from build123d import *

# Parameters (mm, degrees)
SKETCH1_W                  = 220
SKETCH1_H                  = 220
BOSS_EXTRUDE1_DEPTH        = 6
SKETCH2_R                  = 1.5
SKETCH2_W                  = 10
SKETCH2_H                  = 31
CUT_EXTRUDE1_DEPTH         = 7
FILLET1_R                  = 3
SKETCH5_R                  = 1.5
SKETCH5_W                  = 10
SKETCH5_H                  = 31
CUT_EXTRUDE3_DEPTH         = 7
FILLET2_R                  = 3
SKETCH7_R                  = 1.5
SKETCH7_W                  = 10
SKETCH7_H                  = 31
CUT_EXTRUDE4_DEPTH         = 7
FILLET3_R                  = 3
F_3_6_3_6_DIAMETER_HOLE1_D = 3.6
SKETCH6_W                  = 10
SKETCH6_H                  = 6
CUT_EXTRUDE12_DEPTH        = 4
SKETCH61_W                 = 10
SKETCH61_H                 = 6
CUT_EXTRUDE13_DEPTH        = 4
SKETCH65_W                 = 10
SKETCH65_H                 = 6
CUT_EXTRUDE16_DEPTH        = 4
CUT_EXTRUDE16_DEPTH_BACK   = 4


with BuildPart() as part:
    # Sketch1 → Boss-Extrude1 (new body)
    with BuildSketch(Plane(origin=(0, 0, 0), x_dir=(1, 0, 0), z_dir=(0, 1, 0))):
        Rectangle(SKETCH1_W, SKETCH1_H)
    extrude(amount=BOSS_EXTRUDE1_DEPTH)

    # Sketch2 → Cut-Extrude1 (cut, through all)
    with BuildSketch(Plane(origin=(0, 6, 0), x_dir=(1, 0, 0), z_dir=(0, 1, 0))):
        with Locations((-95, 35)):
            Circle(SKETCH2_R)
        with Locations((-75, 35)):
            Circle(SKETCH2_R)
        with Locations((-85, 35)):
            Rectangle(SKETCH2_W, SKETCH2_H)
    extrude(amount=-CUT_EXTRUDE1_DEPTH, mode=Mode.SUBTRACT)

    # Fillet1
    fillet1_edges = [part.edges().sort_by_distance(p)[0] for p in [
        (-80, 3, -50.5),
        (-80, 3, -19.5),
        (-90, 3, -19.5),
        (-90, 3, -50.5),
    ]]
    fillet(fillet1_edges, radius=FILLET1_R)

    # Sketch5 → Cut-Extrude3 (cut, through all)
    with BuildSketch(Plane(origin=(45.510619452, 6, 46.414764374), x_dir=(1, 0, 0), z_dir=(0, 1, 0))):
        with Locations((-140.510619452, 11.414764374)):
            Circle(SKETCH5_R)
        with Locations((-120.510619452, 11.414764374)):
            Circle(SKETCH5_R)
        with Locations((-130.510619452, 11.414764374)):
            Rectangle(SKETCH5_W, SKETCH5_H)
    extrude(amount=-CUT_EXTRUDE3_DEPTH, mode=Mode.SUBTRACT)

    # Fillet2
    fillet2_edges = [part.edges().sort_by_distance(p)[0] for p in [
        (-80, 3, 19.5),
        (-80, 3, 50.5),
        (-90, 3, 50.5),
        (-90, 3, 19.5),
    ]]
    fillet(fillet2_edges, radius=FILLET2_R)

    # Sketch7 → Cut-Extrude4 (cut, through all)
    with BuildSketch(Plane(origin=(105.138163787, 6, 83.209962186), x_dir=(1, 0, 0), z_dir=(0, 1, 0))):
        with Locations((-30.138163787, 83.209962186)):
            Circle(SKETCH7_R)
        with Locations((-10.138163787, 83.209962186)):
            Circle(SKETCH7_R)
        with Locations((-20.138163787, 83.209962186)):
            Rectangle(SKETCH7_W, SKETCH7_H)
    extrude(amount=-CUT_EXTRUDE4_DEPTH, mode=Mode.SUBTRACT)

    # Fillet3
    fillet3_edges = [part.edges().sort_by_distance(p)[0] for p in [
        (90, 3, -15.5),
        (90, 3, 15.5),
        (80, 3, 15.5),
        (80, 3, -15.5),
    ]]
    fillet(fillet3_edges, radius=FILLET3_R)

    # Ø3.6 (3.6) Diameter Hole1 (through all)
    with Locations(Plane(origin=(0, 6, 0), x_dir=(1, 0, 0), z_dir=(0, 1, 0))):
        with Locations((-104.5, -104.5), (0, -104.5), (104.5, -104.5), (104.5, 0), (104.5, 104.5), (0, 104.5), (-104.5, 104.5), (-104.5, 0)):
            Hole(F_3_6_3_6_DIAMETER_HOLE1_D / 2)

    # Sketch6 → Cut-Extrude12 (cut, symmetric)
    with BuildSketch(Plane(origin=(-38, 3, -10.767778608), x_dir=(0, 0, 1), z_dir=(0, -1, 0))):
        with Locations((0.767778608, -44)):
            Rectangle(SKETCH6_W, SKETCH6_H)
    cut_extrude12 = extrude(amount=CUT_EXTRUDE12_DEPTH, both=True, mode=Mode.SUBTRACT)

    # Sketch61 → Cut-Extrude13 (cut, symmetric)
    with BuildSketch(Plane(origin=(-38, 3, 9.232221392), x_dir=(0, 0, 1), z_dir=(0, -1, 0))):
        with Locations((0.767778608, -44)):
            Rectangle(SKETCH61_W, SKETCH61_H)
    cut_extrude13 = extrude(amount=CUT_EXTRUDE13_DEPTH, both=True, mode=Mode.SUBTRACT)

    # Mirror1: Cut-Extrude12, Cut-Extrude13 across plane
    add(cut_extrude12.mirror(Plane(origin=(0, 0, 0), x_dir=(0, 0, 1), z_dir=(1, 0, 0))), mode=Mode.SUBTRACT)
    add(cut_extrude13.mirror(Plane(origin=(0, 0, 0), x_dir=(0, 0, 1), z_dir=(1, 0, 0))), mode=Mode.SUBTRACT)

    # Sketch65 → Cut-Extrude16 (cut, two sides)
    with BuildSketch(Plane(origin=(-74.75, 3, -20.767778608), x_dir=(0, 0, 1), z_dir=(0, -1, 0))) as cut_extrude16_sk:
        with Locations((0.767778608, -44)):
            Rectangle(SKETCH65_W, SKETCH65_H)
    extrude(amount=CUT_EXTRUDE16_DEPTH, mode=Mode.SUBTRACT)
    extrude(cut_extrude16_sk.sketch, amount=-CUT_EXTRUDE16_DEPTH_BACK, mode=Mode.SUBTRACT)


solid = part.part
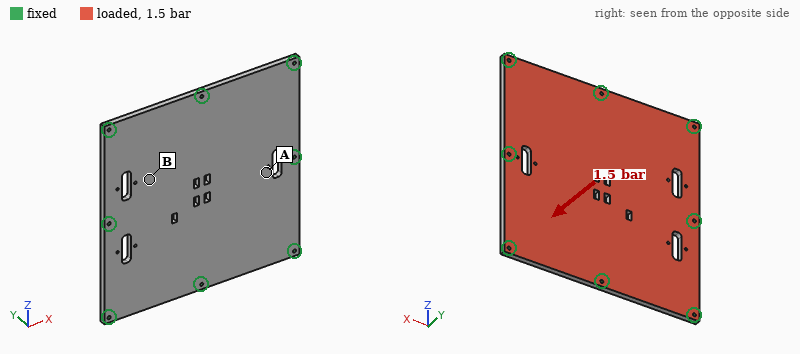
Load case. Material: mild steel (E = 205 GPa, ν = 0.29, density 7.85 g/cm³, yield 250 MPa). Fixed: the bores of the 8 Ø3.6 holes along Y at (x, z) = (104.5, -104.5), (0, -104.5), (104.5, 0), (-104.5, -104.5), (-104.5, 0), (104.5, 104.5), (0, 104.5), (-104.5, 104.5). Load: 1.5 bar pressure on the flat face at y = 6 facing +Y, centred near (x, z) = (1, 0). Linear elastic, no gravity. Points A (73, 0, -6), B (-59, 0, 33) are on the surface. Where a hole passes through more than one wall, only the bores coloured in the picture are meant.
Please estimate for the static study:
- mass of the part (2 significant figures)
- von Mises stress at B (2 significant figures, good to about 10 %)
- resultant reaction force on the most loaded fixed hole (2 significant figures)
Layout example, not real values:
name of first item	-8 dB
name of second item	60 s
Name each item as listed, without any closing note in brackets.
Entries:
mass of the part	2.2 kg
von Mises stress at B	27 MPa
resultant reaction force on the most loaded fixed hole	1.4 kN
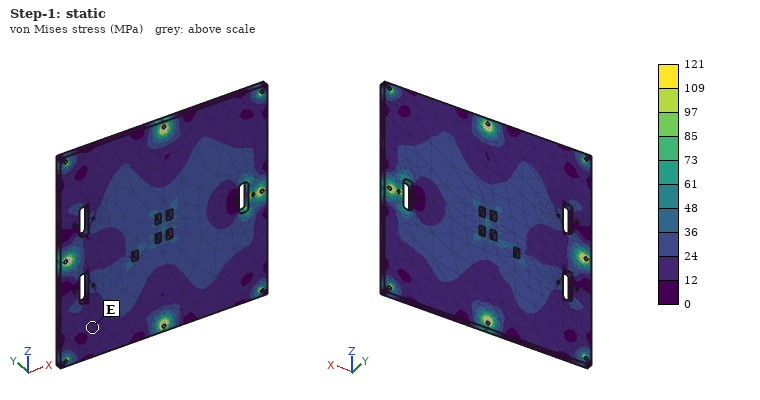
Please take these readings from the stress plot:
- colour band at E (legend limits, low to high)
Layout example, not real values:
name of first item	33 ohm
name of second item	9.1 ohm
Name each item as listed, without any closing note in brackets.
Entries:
colour band at E	12 to 24 MPa
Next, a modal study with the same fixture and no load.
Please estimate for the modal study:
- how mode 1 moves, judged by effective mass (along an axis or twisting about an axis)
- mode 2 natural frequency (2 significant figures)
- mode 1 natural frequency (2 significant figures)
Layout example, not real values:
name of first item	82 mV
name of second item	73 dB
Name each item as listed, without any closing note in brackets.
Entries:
how mode 1 moves, judged by effective mass	along Y
mode 2 natural frequency	1600 Hz
mode 1 natural frequency	870 Hz
